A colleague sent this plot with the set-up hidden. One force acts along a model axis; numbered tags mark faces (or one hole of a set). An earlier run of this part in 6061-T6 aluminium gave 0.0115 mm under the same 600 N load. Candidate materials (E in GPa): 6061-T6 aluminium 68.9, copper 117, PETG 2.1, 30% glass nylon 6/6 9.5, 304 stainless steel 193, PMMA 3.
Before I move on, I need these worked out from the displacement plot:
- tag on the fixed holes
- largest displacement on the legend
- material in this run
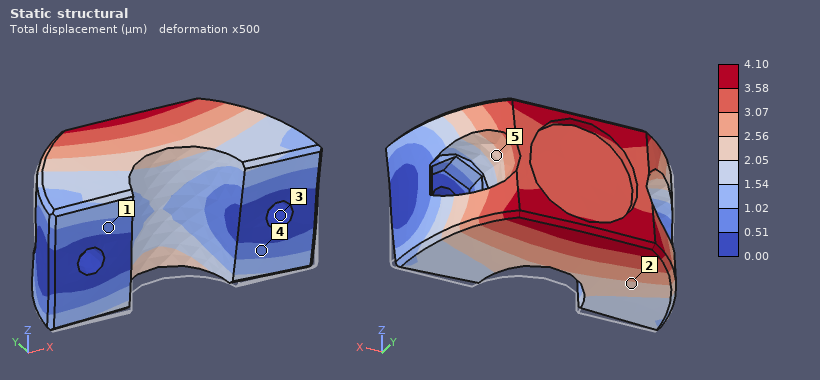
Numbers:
3
4.10 µm
304 stainless steel
